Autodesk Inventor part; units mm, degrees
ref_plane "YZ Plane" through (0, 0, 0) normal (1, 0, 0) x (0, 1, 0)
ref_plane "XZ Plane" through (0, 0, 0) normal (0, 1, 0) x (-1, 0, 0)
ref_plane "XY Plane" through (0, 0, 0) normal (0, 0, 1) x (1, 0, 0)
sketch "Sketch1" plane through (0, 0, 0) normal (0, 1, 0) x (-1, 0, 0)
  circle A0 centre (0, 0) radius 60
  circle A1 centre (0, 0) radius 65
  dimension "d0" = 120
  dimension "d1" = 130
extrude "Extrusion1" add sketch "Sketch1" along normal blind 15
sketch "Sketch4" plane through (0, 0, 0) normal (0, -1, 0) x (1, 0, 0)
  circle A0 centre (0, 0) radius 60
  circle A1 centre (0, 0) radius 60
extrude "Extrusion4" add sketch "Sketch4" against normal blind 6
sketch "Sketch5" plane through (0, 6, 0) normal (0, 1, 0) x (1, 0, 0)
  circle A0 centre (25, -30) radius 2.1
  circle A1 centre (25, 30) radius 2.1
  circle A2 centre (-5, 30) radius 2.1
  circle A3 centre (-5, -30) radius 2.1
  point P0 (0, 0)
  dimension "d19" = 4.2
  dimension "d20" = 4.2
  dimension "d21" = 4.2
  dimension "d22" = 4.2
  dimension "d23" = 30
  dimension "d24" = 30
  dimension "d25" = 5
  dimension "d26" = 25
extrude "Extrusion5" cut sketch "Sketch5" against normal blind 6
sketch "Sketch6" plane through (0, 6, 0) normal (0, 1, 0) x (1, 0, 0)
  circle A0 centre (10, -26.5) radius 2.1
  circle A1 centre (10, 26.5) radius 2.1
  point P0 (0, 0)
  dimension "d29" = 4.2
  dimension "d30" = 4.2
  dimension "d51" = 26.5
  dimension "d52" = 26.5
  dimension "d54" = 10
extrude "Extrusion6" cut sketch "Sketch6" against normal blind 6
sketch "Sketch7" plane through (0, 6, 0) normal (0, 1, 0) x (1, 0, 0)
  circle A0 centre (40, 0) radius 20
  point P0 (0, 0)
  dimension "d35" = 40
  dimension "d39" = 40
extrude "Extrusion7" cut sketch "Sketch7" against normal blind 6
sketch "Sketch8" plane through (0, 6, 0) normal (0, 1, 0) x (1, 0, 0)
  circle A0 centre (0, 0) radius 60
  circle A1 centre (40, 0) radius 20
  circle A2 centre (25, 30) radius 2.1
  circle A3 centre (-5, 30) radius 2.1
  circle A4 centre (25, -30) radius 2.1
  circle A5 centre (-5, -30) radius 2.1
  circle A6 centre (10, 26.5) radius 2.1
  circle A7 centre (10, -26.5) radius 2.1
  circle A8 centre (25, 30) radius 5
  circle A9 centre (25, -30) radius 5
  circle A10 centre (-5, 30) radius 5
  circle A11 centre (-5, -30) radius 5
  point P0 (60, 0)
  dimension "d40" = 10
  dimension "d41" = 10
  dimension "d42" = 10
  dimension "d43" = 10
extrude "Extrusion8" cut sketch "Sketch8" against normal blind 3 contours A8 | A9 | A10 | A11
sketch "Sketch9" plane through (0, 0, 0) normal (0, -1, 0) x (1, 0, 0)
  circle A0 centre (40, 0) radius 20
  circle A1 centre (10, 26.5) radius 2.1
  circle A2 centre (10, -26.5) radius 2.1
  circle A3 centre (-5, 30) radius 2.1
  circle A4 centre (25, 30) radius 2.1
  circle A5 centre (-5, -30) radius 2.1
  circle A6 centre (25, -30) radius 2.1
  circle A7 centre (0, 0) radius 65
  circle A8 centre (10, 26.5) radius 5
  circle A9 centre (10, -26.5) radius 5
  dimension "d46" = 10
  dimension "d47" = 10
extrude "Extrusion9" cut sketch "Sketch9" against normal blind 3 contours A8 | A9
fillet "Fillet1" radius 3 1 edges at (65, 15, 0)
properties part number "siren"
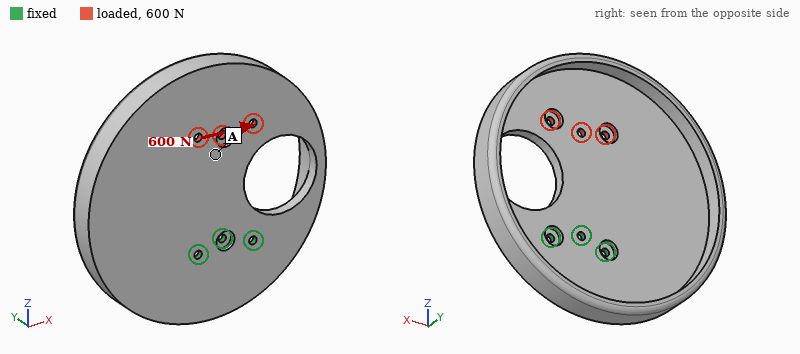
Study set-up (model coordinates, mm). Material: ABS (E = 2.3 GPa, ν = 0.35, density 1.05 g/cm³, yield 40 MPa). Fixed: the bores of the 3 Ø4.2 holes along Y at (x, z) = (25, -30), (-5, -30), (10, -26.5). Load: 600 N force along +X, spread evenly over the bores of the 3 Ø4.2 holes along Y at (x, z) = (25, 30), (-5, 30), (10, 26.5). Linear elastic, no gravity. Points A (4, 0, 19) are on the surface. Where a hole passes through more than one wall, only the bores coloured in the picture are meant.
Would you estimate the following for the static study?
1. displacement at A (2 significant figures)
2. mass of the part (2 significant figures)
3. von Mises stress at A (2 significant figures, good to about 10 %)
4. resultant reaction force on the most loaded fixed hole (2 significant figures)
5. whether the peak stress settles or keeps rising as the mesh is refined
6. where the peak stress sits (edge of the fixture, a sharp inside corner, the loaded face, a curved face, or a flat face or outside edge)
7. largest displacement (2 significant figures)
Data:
0.48 mm
92 g
3.3 MPa
1.1 kN
keeps rising
edge of the fixture
0.92 mm
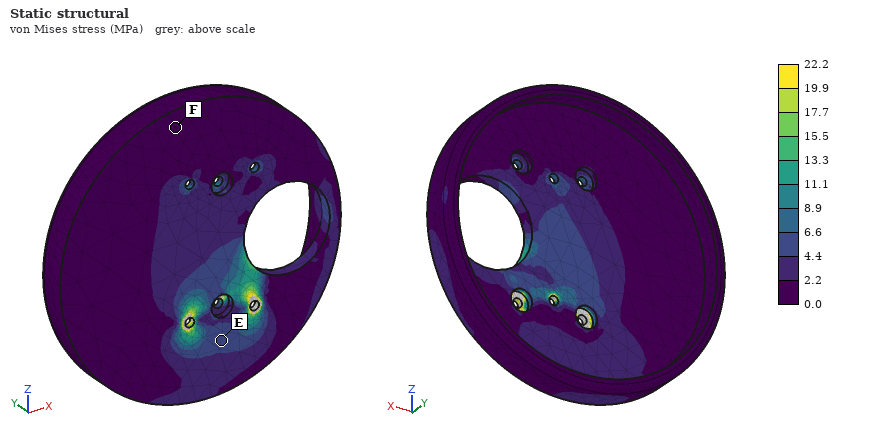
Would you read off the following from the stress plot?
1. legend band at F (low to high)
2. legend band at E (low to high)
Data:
0.0 to 2.2 MPa
4.4 to 6.6 MPa
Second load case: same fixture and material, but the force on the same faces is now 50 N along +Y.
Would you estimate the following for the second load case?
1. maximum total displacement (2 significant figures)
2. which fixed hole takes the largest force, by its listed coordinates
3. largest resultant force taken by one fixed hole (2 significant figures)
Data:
2.0 mm
(10, -26.5)
310 N
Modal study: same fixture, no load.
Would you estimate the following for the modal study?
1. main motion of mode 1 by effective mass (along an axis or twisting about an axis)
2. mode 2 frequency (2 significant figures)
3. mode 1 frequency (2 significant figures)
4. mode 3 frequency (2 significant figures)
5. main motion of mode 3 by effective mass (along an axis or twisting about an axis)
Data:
along Y
300 Hz
130 Hz
580 Hz
along X
